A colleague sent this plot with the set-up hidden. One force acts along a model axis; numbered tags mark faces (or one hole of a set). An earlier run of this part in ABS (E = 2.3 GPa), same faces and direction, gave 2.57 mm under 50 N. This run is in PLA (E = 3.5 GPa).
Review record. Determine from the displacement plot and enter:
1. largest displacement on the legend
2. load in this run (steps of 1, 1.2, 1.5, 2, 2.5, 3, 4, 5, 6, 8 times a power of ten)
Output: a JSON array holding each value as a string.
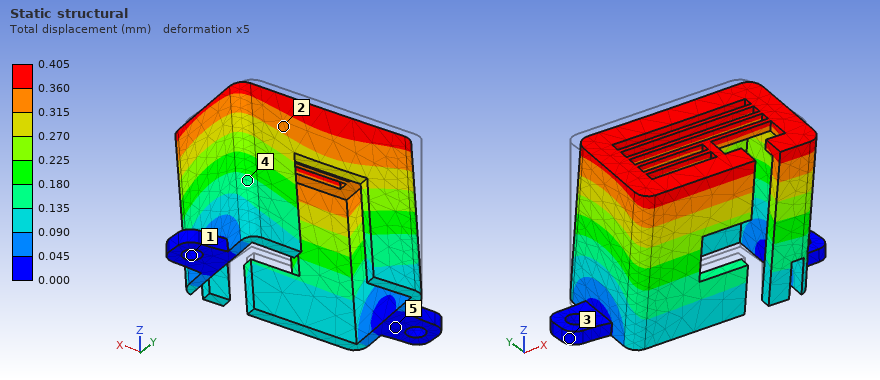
["0.405 mm", "12 N"]
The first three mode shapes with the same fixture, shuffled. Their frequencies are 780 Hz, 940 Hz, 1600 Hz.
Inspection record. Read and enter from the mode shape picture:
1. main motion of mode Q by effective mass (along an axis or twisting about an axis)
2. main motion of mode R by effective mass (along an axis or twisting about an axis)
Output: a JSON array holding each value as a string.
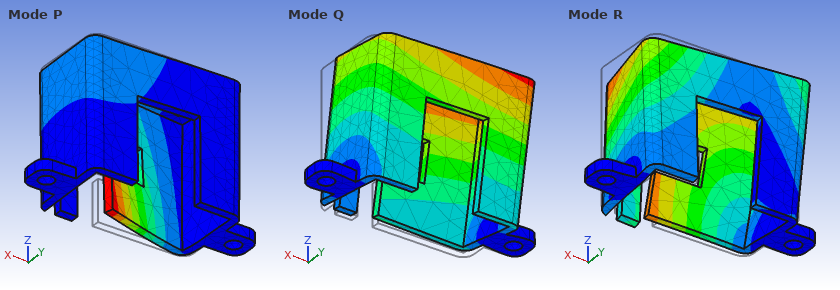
["along Y", "along X"]
